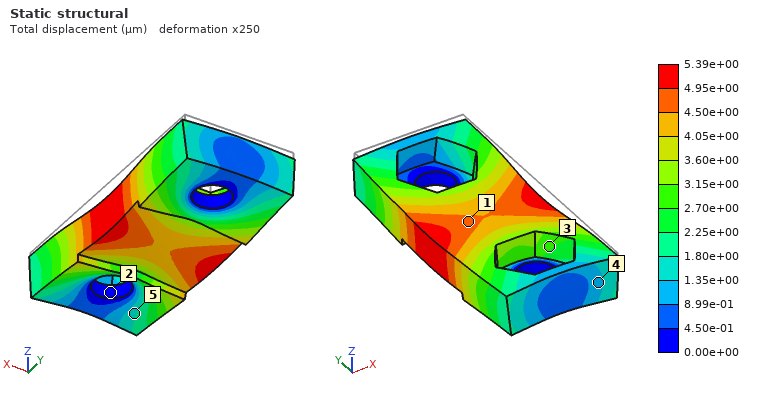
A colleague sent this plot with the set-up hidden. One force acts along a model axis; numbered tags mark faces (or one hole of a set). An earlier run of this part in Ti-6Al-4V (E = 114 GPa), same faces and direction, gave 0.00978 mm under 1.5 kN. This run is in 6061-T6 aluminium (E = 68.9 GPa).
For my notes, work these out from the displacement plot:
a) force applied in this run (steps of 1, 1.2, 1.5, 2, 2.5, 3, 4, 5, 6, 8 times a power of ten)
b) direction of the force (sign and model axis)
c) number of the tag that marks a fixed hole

500 N
-Z
2
